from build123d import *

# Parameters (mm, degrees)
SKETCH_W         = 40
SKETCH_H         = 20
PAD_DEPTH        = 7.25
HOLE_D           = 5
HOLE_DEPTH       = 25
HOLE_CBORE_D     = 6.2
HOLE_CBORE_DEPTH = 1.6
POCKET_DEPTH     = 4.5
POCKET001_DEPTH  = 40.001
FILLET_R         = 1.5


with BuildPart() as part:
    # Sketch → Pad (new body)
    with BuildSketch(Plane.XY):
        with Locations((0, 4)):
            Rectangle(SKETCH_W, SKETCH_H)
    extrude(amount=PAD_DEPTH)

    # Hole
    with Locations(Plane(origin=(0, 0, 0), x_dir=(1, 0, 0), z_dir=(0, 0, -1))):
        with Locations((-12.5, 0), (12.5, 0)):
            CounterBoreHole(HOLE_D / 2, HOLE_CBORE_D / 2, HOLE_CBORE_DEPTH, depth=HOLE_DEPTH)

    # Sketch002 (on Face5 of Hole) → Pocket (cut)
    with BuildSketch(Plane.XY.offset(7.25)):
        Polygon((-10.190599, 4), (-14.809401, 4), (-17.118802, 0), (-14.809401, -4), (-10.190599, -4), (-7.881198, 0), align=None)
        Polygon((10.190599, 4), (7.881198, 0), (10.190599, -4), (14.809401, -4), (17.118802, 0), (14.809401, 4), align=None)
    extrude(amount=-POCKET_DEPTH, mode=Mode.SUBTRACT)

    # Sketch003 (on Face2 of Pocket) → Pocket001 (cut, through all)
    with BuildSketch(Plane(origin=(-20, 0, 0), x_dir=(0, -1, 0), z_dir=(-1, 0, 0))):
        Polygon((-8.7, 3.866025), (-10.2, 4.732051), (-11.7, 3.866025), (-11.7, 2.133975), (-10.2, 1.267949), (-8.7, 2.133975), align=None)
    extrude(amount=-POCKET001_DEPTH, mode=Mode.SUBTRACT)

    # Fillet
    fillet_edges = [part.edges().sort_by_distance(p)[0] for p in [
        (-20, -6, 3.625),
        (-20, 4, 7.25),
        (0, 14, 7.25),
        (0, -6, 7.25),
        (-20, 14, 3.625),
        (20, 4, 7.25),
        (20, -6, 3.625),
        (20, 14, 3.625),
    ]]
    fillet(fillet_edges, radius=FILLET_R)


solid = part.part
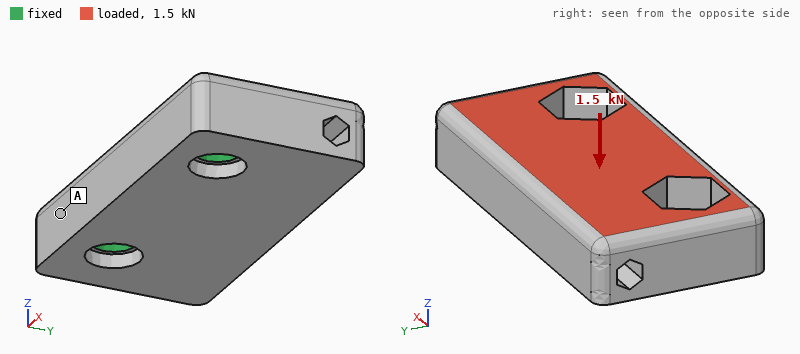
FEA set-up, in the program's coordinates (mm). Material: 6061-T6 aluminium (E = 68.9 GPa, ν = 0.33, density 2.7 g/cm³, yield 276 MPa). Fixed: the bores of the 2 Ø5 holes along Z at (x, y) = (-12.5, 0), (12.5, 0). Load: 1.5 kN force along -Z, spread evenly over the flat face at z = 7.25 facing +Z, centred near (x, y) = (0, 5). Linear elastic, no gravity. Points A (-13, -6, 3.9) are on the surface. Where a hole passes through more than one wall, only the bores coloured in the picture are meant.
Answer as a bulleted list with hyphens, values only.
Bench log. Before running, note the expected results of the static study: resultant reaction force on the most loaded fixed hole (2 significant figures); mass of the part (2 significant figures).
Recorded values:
- 760 N
- 13 g
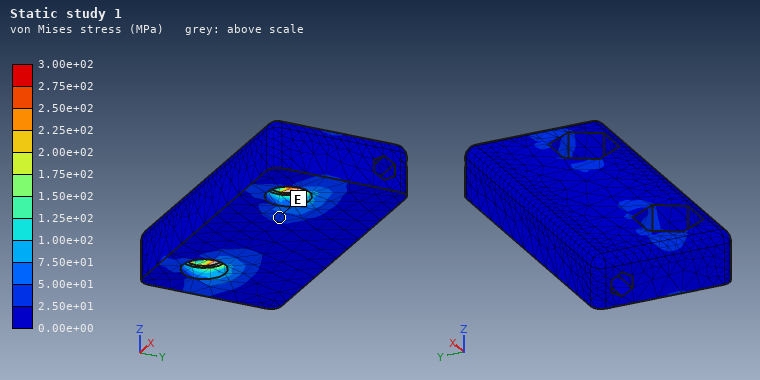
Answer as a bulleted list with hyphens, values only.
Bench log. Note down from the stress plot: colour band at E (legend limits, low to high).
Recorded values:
- 2.50e+01 to 5.00e+01 MPa
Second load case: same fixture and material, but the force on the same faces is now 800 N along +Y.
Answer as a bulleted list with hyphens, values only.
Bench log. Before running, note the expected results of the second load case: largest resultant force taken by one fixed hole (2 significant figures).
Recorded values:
- 400 N
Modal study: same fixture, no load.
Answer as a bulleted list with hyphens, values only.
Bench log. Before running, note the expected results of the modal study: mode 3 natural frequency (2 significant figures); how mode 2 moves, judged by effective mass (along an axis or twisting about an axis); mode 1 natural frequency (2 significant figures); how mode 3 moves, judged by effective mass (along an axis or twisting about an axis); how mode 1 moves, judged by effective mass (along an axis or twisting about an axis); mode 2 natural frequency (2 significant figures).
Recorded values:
- 24 kHz
- twisting about Y
- 8000 Hz
- along Z
- along Z
- 19 kHz
